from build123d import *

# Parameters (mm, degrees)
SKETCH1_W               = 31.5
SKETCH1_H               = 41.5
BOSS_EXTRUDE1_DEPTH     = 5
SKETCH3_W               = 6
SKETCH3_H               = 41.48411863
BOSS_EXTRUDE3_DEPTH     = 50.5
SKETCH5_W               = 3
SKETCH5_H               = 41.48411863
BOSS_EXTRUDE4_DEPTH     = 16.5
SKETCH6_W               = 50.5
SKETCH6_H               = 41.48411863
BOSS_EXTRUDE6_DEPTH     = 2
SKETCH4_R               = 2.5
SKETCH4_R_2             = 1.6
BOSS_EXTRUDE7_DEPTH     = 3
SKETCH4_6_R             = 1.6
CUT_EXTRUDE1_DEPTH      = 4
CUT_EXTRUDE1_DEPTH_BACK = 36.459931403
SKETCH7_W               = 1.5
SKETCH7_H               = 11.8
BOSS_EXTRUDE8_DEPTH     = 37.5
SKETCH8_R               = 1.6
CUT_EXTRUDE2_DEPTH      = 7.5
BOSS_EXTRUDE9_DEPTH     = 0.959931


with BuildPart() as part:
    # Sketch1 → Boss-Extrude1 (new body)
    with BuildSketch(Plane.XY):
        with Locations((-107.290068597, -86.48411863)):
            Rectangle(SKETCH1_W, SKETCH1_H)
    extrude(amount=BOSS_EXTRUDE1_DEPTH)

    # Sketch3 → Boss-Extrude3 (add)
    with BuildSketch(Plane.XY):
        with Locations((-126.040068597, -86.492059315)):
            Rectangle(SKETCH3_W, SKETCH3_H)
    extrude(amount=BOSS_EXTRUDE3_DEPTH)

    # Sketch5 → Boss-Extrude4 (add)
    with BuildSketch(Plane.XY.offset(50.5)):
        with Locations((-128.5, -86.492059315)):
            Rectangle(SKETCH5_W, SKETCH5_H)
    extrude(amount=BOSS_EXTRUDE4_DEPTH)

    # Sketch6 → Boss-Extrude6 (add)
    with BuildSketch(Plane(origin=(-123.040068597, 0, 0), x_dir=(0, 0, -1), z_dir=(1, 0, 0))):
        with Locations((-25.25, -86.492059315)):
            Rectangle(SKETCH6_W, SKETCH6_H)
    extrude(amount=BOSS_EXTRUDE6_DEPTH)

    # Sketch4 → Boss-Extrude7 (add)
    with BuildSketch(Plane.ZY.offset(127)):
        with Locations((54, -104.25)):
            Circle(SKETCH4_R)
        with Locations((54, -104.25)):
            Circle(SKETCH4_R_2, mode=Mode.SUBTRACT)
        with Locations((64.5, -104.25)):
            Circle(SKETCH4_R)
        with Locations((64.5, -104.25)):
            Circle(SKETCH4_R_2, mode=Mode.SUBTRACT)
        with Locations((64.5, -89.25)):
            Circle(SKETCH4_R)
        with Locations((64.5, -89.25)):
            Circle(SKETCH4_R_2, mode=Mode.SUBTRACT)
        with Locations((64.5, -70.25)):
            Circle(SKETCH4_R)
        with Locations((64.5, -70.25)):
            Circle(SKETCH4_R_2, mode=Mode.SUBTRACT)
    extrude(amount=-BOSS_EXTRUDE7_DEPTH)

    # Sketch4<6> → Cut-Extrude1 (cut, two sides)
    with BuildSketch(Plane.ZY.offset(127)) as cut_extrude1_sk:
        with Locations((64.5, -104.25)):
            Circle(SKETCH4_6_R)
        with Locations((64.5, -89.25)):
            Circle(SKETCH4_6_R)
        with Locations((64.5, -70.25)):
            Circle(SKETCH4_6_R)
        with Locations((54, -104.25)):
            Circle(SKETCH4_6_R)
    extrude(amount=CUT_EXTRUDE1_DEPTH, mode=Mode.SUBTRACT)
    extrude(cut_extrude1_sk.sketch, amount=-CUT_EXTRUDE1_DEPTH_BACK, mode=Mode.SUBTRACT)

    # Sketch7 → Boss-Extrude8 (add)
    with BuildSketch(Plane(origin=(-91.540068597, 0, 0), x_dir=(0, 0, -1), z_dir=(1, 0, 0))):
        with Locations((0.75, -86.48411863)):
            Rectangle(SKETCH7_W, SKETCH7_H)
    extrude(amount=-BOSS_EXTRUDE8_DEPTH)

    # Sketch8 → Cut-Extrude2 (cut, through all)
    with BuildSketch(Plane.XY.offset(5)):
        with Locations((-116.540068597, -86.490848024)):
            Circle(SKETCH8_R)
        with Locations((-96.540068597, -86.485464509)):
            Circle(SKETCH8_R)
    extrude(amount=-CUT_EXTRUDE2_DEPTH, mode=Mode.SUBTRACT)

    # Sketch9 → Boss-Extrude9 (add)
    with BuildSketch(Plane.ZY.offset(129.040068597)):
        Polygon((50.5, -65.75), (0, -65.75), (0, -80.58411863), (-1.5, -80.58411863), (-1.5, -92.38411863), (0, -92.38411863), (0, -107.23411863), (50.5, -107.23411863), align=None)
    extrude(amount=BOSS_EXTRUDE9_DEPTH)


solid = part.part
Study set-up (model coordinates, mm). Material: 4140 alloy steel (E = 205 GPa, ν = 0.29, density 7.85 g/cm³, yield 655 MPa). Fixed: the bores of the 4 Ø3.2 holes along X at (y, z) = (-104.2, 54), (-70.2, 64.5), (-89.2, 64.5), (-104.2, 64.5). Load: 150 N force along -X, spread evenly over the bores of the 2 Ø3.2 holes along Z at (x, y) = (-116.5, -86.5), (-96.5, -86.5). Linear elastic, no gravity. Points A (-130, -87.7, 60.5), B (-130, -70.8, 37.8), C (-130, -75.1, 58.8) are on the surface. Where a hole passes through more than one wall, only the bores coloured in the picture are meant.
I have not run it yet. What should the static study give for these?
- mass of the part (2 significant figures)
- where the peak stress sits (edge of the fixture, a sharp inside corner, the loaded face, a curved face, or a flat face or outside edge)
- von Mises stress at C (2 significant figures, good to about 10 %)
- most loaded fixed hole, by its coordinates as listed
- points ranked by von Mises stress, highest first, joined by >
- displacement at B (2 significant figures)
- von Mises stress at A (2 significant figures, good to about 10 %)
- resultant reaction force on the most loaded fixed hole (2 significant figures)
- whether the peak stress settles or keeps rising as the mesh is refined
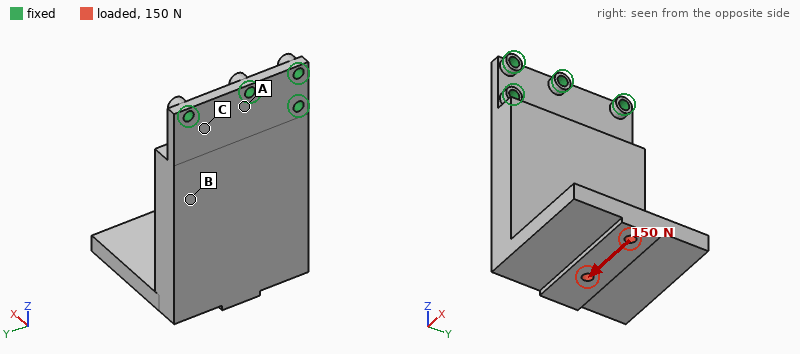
220 g
edge of the fixture
68 MPa
(-104.2, 54)
C > A > B
0.069 mm
52 MPa
310 N
keeps rising
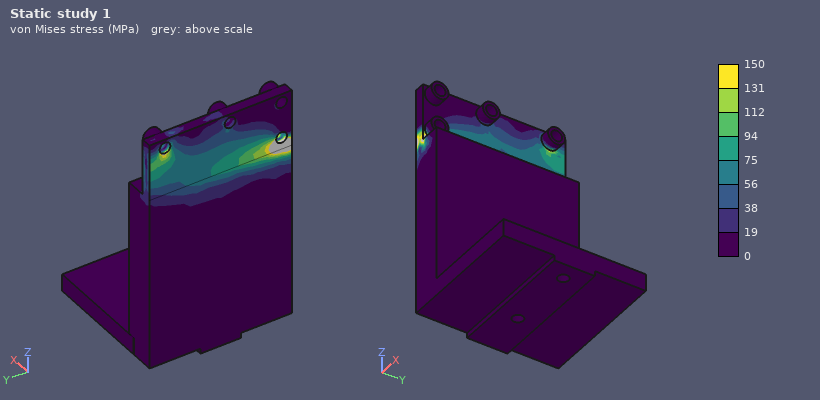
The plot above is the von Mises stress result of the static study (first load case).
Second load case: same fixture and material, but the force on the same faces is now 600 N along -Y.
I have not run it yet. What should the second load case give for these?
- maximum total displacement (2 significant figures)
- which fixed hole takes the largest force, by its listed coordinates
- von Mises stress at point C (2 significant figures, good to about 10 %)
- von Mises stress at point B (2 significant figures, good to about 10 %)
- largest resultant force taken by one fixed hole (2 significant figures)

0.12 mm
(-104.2, 54)
56 MPa
15 MPa
1.1 kN
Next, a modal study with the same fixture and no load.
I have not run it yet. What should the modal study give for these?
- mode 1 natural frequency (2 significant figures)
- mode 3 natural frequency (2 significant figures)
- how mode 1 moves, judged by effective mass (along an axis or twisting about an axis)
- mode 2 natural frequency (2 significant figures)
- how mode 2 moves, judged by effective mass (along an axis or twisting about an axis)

410 Hz
3500 Hz
along X
2200 Hz
along Y
